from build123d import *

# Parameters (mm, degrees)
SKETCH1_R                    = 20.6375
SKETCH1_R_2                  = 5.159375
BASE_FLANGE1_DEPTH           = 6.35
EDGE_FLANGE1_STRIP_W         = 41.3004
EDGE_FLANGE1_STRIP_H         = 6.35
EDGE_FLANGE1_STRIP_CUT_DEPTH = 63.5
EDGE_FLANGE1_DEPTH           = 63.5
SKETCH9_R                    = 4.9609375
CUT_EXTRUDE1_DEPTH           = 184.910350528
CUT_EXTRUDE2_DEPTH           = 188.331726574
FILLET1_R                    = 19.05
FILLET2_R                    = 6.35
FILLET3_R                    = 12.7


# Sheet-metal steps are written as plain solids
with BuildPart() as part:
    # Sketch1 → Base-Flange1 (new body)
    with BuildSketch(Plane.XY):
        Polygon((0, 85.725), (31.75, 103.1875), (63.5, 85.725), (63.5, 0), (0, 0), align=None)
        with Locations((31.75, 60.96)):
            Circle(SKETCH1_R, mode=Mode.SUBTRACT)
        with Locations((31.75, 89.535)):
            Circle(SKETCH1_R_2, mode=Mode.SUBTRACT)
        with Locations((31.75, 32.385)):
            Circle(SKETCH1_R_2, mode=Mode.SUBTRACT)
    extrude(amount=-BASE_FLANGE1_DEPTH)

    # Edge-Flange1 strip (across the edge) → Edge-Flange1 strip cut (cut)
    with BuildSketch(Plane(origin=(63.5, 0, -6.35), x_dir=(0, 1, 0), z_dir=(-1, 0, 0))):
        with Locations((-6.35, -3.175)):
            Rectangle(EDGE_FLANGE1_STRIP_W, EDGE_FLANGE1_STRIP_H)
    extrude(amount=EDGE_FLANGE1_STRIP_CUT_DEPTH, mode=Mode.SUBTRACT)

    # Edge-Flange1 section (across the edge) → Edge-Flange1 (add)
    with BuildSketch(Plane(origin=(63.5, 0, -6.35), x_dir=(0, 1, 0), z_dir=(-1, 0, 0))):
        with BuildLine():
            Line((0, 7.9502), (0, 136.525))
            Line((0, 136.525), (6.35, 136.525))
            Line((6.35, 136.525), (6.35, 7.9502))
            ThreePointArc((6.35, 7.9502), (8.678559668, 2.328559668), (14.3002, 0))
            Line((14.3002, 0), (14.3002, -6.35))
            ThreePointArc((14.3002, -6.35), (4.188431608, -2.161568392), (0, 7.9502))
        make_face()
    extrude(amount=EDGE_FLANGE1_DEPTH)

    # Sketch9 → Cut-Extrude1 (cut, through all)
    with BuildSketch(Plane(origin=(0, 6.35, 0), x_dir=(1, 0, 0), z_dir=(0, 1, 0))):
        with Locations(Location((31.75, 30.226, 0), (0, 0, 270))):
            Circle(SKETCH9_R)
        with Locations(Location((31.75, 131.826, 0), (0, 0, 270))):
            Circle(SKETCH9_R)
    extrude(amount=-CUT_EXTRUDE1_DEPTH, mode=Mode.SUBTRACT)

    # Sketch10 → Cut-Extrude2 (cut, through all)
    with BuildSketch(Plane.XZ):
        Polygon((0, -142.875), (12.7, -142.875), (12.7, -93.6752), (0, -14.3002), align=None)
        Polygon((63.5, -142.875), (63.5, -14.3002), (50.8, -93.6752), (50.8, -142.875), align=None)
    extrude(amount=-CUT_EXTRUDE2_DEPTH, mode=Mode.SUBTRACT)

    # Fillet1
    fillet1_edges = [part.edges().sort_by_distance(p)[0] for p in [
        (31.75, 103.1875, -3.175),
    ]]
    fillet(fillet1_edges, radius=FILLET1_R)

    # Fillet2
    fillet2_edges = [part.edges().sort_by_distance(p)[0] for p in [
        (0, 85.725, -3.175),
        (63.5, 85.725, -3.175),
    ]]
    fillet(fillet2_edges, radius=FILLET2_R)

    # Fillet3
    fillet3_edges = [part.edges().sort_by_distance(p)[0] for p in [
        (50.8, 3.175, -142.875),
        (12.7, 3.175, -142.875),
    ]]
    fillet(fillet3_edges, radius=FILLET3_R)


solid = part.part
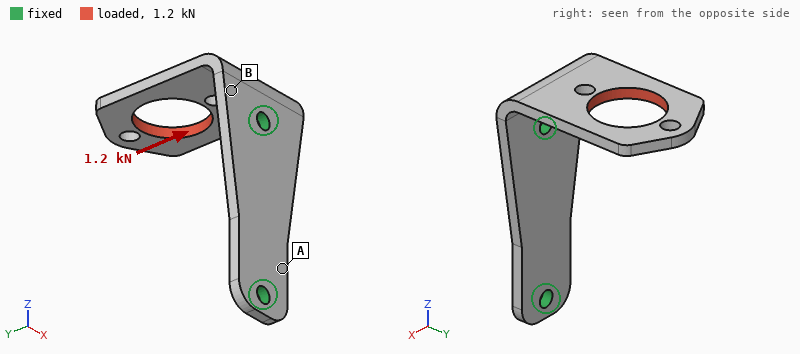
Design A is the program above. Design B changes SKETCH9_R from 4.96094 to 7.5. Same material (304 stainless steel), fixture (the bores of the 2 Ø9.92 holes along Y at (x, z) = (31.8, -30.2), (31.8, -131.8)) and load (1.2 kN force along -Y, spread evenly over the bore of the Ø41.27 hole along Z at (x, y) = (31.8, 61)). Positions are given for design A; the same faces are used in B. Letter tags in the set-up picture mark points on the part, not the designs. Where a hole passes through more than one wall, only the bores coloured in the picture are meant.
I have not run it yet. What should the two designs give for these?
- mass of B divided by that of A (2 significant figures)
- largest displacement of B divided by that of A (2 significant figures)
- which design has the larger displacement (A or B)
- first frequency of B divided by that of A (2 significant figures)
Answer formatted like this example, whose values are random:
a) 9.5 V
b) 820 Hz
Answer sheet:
a) 0.98
b) 0.77
c) A
d) 1.0
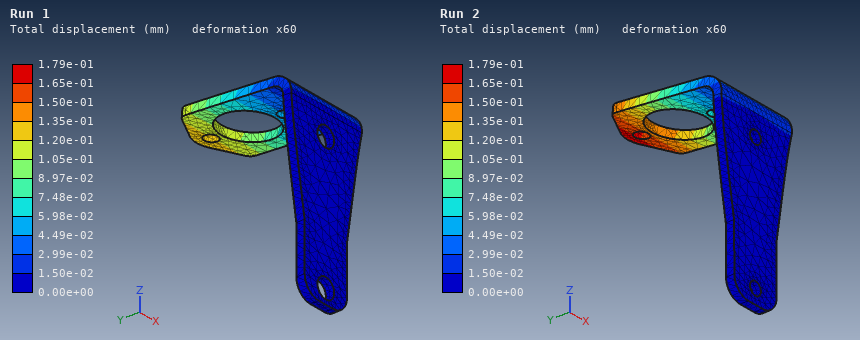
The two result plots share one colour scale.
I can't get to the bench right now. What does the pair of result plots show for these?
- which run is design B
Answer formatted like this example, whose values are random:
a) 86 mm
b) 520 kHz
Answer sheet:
a) Run 1
